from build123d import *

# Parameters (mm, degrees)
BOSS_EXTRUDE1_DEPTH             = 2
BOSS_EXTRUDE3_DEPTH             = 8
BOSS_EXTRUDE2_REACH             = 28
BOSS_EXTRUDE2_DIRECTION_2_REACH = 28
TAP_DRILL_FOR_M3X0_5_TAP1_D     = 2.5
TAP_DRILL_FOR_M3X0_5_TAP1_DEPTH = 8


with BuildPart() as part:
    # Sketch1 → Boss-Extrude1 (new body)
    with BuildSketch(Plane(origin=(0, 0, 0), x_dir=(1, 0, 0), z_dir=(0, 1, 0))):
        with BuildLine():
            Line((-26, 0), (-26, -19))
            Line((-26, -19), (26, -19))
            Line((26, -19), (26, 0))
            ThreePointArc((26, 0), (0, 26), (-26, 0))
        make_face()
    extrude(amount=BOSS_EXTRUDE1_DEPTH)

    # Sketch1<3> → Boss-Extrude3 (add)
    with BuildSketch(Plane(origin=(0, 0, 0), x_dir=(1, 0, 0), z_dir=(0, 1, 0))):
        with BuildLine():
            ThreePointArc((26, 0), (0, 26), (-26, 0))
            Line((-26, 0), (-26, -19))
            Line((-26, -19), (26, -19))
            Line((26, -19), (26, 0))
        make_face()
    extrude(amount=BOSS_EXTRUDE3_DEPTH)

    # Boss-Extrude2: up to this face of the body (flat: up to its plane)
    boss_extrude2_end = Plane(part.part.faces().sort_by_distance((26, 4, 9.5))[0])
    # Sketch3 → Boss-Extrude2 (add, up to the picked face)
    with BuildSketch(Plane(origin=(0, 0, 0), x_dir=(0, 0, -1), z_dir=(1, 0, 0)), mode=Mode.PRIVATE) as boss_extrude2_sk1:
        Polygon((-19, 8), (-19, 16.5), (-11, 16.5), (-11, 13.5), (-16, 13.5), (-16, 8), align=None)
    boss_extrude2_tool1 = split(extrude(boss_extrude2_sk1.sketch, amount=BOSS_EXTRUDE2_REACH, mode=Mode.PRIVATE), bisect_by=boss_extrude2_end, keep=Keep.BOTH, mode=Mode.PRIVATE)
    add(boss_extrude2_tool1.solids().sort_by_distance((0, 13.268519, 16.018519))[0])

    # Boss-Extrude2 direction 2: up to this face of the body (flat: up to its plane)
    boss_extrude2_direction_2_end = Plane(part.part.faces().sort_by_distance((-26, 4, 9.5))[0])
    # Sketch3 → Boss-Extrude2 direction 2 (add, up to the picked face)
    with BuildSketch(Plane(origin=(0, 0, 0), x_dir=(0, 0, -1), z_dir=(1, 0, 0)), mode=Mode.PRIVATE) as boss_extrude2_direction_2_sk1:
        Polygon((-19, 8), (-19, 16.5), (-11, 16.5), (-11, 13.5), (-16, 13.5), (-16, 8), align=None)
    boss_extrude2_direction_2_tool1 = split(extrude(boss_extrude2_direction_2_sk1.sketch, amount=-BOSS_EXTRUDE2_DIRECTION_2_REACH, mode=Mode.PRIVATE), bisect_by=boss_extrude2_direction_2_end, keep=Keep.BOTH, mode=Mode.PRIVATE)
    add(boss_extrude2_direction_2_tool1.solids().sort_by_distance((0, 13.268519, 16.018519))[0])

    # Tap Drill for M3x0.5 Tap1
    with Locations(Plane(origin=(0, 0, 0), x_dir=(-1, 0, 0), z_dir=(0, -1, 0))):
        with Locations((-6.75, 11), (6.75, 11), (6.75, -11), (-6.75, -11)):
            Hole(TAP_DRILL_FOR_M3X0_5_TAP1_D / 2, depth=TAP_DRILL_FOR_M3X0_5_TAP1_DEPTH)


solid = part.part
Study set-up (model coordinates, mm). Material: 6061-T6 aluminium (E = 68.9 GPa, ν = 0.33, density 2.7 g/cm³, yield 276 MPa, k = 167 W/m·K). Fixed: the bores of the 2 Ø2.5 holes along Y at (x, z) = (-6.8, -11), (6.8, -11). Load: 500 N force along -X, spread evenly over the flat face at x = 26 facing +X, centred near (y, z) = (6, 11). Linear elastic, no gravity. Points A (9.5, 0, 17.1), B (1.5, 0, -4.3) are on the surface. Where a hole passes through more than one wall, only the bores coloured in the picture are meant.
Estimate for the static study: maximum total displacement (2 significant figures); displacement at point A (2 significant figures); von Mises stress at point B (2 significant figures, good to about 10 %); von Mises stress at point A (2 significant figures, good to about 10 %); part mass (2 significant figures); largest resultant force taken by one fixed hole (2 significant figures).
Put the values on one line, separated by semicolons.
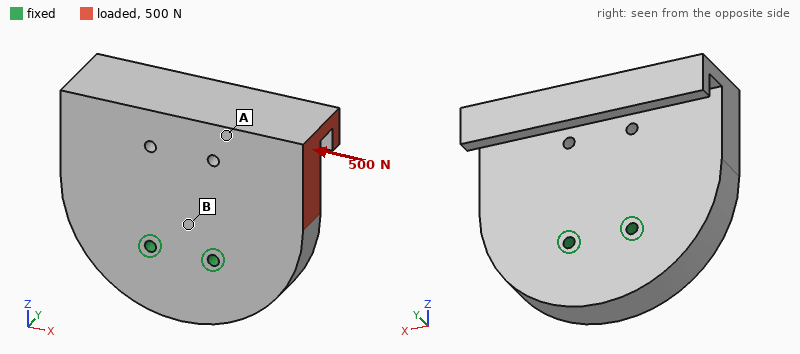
10 µm; 5.9 µm; 5.8 MPa; 2.8 MPa; 50 g; 770 N
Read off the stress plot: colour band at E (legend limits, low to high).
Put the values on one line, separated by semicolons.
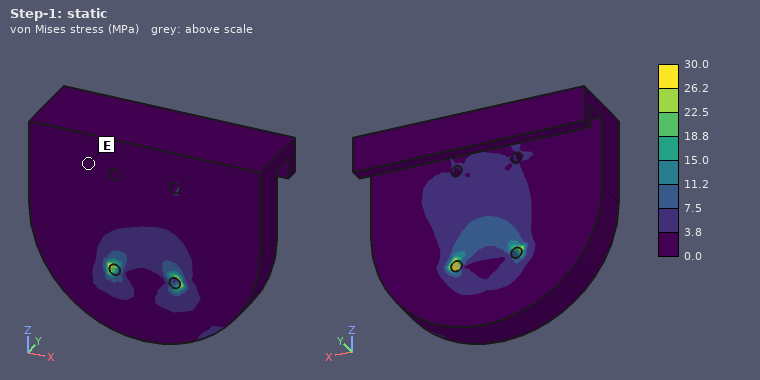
0.0 to 3.8 MPa
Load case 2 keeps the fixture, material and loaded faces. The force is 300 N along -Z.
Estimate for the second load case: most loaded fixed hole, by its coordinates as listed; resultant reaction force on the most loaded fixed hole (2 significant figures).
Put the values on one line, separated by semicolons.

(6.8, -11); 670 N
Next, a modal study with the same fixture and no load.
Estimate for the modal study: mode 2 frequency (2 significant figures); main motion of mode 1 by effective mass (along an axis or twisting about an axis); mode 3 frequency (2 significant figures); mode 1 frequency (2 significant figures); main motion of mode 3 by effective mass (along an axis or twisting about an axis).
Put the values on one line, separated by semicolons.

6000 Hz; along Y; 8200 Hz; 4200 Hz; along X
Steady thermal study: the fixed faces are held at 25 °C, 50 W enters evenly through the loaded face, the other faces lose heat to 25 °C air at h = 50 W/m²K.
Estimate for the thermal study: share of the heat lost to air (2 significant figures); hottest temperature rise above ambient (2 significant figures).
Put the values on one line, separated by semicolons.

9.3 %; 45 K
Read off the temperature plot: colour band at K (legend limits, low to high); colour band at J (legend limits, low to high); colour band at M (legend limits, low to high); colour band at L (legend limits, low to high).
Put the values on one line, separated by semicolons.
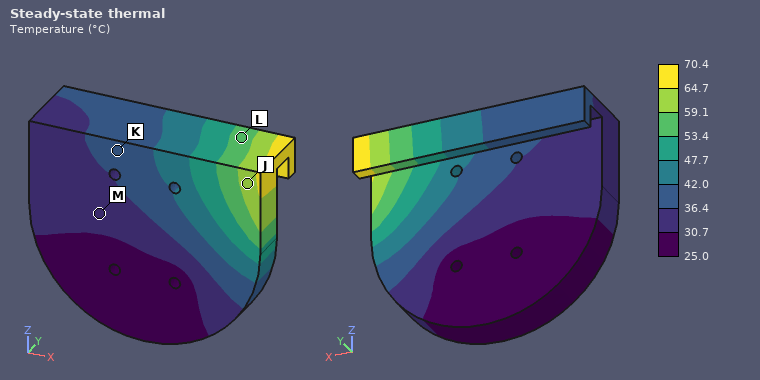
36.4 to 42.0 °C; 59.1 to 64.7 °C; 30.7 to 36.4 °C; 53.4 to 59.1 °C
